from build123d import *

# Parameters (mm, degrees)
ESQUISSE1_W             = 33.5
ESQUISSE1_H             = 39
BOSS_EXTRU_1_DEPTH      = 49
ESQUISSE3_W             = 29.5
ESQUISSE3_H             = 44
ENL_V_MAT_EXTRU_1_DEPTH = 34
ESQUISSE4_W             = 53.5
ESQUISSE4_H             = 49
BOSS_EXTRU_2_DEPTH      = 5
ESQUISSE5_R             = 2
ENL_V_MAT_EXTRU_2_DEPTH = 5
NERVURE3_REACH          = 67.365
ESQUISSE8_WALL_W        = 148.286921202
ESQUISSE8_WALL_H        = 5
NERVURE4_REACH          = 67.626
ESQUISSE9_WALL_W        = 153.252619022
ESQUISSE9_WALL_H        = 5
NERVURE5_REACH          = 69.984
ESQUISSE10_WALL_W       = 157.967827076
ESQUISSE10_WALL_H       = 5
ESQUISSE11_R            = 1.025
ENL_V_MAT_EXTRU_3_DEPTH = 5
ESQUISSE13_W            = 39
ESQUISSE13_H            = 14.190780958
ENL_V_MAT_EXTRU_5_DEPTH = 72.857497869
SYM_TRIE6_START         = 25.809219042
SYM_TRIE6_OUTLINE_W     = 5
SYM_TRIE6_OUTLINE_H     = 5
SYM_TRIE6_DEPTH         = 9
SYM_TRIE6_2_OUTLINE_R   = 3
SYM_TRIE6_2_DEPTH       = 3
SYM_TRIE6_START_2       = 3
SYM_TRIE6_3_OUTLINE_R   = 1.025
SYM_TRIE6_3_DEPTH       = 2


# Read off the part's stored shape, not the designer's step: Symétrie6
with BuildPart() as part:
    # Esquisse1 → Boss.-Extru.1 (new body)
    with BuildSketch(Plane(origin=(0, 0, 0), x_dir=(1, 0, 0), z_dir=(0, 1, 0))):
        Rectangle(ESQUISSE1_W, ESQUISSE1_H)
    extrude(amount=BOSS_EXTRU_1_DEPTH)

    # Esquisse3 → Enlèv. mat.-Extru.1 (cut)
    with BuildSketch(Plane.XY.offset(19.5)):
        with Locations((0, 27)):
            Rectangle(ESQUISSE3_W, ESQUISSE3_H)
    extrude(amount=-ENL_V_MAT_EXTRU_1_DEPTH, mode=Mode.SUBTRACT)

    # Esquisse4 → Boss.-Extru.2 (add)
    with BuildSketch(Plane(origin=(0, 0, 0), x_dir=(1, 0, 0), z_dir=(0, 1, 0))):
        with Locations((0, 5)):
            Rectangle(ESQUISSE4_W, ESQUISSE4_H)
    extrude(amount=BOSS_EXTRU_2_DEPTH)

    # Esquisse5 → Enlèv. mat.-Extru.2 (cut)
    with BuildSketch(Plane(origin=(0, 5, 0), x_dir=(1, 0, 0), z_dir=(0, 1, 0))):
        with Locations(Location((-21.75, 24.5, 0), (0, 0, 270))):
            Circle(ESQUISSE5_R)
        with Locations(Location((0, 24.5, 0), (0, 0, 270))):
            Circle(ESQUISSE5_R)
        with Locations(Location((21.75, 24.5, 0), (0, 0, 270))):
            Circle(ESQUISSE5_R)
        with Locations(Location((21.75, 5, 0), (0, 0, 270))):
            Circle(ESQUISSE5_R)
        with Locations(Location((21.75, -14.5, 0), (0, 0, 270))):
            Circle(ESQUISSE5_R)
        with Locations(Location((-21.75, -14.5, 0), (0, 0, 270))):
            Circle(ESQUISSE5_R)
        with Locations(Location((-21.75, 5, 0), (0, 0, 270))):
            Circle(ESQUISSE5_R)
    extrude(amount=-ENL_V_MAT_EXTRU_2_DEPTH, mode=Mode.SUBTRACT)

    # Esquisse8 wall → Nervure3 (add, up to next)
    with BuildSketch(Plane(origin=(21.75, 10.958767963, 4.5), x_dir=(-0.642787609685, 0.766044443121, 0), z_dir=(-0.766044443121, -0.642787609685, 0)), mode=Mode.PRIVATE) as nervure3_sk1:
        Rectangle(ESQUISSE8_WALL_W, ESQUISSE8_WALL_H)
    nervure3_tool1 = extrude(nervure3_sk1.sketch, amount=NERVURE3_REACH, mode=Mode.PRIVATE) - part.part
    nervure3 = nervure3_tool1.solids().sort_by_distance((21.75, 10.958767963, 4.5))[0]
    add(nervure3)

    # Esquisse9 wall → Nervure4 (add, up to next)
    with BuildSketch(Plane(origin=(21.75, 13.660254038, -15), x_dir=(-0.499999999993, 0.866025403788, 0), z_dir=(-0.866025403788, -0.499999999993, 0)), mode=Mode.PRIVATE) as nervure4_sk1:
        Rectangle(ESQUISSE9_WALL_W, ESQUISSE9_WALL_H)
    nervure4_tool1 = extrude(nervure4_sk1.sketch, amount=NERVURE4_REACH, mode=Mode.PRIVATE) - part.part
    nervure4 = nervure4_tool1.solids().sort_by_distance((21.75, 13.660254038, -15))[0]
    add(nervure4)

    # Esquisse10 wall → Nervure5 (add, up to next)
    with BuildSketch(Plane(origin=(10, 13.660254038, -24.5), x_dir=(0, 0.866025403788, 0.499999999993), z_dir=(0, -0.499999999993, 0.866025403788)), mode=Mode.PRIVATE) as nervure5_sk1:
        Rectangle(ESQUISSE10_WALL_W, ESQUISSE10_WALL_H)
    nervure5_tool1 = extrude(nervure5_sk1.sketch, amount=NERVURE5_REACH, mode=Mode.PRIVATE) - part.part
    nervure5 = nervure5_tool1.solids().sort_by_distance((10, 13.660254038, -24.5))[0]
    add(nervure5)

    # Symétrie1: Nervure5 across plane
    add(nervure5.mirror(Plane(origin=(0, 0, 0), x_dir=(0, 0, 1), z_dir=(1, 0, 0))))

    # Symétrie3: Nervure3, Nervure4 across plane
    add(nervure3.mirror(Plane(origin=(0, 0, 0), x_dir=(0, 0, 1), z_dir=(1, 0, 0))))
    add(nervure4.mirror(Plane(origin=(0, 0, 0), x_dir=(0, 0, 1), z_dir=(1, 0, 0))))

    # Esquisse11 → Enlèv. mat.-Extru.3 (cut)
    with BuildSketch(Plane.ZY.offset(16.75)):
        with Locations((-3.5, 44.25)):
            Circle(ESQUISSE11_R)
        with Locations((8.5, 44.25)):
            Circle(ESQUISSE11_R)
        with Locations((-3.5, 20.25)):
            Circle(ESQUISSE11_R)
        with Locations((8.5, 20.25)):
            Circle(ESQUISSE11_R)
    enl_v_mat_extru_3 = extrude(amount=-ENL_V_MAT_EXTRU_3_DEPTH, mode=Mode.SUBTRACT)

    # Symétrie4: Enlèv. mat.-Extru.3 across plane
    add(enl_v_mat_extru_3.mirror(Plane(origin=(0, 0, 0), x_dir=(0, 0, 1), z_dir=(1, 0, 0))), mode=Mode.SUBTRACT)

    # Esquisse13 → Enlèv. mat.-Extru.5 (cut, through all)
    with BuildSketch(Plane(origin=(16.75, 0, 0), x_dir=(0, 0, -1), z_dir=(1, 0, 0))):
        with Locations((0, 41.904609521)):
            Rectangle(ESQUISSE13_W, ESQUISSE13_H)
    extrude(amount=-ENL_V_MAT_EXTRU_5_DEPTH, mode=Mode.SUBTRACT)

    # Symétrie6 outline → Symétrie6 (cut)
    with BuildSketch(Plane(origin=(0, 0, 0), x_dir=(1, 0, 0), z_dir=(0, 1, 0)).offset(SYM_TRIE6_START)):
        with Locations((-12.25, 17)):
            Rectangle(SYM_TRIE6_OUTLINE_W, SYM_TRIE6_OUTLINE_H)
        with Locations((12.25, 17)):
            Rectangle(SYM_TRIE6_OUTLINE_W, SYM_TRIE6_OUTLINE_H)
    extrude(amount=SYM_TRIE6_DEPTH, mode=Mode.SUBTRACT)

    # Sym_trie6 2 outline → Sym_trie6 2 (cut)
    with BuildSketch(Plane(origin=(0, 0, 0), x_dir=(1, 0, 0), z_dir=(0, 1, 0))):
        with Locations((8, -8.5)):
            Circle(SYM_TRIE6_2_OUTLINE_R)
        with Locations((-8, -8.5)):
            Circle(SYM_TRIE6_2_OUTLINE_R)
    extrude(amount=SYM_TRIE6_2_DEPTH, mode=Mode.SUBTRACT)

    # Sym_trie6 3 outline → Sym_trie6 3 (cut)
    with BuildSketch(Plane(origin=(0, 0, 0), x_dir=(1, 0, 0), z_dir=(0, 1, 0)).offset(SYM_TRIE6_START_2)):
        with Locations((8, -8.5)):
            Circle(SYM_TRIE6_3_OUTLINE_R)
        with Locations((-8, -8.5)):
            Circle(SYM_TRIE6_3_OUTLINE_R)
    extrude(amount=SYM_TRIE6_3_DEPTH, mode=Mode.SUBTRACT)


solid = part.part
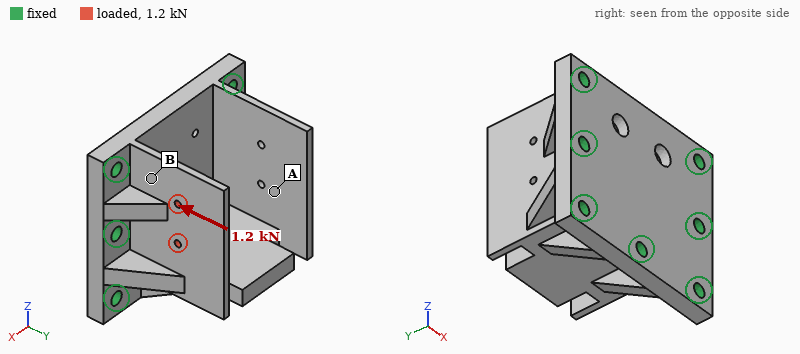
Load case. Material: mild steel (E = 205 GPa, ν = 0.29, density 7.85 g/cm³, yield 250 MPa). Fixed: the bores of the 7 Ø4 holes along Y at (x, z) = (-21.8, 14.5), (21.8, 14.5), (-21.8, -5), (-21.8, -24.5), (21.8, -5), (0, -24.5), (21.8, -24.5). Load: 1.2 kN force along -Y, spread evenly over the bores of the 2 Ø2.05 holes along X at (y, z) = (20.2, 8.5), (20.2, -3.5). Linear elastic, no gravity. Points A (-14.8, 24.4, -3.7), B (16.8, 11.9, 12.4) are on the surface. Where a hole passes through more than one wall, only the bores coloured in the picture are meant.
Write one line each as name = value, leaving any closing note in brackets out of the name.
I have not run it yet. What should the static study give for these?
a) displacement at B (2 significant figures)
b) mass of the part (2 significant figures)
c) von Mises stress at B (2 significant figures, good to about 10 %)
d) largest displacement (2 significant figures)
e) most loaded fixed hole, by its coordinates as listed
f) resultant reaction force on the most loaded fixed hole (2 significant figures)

displacement at B = 2.5 µm
mass of the part = 180 g
von Mises stress at B = 19 MPa
largest displacement = 8.3 µm
most loaded fixed hole, by its coordinates as listed = (21.8, 14.5)
resultant reaction force on the most loaded fixed hole = 550 N
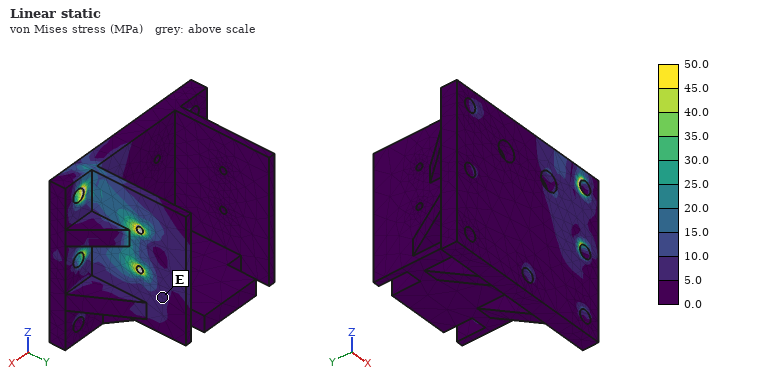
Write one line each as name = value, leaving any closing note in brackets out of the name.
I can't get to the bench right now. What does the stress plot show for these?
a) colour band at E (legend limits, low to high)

colour band at E = 5.0 to 10.0 MPa
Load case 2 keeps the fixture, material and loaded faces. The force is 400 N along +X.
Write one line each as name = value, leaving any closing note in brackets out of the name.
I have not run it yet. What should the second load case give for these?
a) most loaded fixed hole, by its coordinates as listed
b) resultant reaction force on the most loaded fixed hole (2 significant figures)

most loaded fixed hole, by its coordinates as listed = (21.8, -5)
resultant reaction force on the most loaded fixed hole = 190 N
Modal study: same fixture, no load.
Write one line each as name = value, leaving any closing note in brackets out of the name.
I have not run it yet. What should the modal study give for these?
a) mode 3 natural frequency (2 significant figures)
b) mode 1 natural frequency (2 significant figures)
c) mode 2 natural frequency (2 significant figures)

mode 3 natural frequency = 8700 Hz
mode 1 natural frequency = 3800 Hz
mode 2 natural frequency = 3900 Hz
